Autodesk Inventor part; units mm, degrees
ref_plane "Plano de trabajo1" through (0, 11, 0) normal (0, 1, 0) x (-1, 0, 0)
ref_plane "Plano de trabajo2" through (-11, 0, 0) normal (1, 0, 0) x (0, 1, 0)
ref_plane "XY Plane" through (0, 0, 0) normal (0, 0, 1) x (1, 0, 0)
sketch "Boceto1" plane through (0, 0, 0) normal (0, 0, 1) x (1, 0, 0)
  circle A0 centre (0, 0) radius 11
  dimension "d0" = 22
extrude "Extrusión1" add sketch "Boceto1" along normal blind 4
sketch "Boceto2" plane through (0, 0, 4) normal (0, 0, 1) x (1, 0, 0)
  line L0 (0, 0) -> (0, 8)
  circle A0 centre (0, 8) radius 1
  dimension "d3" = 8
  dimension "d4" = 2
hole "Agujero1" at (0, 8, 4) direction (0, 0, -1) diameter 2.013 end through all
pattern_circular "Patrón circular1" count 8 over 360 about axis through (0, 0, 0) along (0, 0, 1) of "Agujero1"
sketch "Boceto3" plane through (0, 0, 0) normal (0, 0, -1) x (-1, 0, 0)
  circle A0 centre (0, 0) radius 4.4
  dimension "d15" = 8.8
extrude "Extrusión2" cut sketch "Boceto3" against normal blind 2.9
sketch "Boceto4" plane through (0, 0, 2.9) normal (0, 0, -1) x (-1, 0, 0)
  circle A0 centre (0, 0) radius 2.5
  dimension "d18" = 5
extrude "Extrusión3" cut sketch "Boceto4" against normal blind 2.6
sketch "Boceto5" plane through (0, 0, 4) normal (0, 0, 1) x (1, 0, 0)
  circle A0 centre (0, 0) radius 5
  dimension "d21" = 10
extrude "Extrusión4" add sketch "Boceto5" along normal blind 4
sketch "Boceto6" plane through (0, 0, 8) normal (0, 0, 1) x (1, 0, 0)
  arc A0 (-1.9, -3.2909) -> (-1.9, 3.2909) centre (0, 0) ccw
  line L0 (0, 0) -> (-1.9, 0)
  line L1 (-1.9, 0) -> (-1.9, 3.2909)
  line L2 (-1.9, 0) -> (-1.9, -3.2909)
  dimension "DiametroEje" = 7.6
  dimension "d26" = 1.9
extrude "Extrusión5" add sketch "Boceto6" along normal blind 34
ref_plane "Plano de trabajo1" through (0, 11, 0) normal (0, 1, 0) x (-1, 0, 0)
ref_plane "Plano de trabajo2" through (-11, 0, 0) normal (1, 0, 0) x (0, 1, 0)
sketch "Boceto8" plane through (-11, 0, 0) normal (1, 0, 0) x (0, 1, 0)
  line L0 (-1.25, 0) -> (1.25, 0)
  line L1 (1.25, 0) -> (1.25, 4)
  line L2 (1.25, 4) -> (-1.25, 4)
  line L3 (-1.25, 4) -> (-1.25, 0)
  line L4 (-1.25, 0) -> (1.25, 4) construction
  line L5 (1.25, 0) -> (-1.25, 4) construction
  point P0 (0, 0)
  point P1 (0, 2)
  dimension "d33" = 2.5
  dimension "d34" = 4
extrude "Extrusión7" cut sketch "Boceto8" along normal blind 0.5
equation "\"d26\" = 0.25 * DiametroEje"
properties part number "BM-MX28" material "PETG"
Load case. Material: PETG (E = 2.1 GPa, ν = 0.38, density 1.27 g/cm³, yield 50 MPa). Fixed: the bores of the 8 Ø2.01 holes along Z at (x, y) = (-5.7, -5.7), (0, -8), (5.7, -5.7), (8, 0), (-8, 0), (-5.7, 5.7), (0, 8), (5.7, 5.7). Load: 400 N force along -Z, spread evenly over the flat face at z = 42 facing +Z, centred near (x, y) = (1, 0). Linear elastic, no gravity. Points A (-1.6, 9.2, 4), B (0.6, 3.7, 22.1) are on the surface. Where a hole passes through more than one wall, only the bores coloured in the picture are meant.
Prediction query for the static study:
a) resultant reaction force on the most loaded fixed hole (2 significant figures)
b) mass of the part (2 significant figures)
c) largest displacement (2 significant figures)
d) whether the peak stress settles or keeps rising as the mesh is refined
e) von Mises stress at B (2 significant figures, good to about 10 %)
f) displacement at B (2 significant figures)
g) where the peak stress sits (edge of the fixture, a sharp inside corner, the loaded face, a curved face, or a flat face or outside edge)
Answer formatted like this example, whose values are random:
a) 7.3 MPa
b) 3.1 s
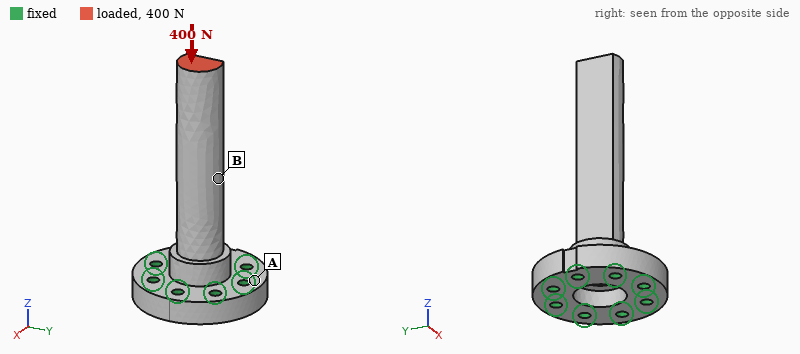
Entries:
a) 75 N
b) 3.5 g
c) 0.23 mm
d) keeps rising
e) 11 MPa
f) 0.11 mm
g) edge of the fixture
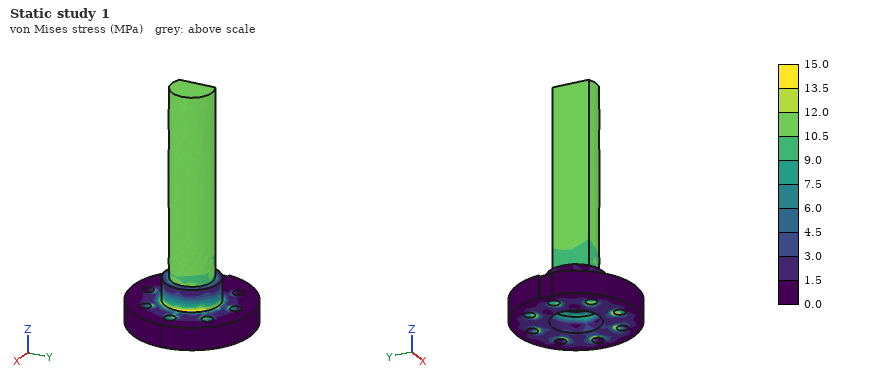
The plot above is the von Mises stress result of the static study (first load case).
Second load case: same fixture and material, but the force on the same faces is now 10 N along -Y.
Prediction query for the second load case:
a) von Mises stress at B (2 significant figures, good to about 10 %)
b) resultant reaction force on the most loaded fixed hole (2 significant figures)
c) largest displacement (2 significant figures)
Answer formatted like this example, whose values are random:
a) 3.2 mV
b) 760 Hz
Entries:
a) 5.2 MPa
b) 17 N
c) 0.59 mm
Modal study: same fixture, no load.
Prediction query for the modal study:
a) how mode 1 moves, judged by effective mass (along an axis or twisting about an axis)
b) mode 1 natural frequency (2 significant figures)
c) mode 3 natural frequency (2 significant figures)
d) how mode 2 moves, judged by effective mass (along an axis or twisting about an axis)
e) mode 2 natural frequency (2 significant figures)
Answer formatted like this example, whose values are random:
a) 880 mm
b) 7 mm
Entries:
a) along X
b) 810 Hz
c) 4600 Hz
d) along Y
e) 1000 Hz
